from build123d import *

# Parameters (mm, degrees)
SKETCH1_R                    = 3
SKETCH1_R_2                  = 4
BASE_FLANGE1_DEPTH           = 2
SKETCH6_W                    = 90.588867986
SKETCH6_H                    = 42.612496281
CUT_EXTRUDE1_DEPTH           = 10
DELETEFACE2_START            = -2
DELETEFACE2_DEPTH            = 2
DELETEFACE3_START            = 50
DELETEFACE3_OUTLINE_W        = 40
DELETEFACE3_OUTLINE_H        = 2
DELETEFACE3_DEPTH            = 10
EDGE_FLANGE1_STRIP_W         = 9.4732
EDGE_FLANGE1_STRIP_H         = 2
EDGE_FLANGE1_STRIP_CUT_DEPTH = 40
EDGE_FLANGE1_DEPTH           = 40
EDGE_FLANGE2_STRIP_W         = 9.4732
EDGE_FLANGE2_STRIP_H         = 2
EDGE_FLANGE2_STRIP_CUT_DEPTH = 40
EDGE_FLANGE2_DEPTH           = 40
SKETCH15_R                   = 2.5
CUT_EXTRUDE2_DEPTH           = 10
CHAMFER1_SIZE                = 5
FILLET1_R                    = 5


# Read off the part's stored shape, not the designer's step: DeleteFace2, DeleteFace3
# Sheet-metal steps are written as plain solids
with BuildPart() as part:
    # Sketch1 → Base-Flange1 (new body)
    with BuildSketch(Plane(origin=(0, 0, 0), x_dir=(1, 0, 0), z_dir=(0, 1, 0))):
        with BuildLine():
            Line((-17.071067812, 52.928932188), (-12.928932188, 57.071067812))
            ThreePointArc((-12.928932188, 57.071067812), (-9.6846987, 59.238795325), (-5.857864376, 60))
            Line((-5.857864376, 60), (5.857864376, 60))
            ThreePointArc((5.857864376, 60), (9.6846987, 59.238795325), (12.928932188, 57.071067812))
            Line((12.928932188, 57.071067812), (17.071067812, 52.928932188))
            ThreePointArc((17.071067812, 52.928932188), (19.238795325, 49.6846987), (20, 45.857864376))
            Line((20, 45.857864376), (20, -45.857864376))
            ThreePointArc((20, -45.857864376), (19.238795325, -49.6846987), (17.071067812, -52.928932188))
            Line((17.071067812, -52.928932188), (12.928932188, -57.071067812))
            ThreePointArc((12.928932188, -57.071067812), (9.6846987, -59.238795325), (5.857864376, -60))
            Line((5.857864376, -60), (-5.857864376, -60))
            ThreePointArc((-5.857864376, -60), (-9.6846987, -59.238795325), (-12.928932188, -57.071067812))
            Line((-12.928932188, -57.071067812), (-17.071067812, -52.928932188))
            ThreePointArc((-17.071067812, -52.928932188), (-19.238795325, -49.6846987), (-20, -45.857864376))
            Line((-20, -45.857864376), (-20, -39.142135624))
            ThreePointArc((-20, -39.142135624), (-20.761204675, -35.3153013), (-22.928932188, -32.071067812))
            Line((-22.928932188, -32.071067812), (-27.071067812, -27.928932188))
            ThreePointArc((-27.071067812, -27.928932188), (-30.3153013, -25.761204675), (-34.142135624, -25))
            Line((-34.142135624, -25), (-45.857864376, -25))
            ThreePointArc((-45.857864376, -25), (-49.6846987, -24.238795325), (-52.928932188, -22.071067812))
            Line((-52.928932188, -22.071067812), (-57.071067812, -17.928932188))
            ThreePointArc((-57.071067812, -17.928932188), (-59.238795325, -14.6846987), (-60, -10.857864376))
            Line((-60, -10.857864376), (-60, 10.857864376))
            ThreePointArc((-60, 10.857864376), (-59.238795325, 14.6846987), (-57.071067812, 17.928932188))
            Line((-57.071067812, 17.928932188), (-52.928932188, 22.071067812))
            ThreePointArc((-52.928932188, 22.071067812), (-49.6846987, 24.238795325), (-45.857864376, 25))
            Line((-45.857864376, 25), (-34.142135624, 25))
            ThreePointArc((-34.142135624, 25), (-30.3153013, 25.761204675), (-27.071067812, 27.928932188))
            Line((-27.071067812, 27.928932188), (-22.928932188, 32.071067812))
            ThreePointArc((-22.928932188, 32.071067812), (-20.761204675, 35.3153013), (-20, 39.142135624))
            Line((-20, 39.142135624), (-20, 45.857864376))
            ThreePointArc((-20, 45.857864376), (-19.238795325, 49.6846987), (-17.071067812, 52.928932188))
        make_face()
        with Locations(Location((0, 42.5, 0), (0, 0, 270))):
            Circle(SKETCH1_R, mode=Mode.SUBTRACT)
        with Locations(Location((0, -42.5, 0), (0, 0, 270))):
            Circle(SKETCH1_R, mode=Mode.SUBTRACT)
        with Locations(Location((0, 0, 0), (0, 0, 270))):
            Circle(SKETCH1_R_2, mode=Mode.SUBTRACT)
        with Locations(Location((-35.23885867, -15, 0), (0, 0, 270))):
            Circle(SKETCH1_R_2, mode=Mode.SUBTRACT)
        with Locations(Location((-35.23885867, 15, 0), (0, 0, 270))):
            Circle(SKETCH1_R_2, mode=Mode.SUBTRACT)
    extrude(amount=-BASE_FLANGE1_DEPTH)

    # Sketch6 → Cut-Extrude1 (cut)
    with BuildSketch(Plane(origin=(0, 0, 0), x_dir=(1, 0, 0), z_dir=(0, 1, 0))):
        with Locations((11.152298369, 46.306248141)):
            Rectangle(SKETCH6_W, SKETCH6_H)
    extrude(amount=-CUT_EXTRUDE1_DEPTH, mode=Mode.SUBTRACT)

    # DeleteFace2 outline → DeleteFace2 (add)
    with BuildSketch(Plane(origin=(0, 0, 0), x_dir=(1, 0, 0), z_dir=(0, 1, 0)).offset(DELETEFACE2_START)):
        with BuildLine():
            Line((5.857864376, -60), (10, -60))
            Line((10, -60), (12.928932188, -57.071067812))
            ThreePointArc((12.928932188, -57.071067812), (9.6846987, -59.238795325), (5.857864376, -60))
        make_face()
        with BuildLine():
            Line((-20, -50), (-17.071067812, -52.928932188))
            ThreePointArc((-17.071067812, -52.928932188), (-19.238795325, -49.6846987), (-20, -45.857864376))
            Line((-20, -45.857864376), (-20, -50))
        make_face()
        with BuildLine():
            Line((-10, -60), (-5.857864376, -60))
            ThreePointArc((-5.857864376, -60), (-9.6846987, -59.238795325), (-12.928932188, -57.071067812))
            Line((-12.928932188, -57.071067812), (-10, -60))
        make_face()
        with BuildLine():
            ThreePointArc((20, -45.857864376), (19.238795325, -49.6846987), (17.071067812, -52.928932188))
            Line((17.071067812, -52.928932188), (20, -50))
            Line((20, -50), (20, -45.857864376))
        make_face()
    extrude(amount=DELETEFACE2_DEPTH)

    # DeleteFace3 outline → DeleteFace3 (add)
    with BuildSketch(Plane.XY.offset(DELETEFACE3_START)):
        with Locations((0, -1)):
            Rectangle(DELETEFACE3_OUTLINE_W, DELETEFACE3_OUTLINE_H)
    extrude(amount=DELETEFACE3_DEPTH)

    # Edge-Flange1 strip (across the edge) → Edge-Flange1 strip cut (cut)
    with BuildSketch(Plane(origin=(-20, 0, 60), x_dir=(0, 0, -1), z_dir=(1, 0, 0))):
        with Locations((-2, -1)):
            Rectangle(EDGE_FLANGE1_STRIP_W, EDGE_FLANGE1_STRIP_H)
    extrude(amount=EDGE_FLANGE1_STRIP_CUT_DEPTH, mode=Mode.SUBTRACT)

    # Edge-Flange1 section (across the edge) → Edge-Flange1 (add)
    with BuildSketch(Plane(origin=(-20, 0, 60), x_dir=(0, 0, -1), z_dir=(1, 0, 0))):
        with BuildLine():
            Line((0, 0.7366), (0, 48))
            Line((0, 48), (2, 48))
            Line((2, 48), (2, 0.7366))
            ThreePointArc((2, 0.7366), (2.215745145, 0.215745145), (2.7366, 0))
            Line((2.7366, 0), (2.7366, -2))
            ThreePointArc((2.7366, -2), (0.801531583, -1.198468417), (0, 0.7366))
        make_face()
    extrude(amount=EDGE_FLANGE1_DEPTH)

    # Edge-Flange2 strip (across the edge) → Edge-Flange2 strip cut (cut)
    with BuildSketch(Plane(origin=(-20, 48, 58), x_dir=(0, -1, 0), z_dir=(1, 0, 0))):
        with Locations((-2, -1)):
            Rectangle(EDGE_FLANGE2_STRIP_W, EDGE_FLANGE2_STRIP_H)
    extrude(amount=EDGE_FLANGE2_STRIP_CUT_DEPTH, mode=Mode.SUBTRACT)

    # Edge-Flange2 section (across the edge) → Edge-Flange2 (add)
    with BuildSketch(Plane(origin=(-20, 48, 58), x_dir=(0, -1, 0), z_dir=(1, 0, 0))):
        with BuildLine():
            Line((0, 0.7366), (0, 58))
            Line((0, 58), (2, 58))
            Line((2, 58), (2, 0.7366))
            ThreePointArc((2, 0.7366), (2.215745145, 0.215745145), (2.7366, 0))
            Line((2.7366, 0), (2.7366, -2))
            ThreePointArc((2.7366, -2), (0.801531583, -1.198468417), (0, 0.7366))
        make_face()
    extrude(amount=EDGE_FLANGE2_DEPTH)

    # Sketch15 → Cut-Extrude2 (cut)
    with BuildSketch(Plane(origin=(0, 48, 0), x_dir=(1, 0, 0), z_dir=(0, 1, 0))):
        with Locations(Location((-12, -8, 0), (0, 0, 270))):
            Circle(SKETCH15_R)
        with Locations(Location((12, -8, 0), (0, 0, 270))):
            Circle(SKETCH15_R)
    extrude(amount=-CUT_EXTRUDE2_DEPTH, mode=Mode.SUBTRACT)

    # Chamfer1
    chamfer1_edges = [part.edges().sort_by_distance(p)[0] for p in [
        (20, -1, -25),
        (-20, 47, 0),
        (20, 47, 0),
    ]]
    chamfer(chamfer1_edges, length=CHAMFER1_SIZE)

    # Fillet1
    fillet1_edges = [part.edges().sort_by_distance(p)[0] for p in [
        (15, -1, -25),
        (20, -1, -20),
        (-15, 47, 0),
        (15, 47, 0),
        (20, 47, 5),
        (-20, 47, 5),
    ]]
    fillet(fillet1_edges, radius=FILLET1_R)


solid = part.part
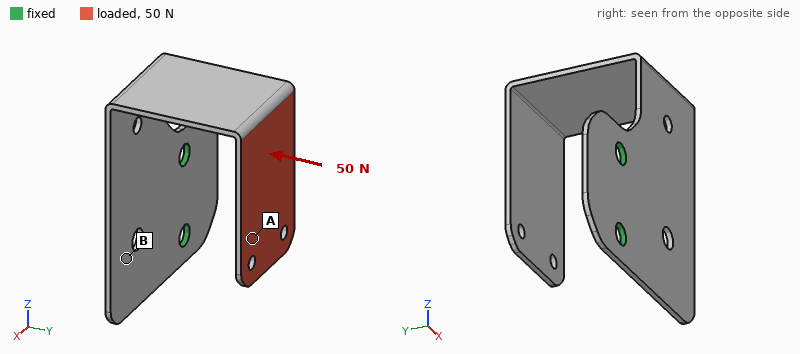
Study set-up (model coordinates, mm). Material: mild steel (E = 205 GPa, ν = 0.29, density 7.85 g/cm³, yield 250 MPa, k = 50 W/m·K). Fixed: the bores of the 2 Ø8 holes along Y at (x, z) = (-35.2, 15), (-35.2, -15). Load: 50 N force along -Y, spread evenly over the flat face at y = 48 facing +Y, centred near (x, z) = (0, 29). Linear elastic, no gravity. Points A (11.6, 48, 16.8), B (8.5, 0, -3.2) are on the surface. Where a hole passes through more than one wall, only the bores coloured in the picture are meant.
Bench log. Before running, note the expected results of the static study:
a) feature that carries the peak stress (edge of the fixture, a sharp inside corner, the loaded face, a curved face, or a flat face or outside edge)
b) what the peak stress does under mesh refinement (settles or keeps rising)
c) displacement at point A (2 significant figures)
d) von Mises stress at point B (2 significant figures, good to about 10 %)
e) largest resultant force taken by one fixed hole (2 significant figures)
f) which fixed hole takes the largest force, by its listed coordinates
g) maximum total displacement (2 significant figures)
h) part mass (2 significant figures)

edge of the fixture
keeps rising
1.0 mm
16 MPa
61 N
(-35.2, 15)
1.3 mm
150 g
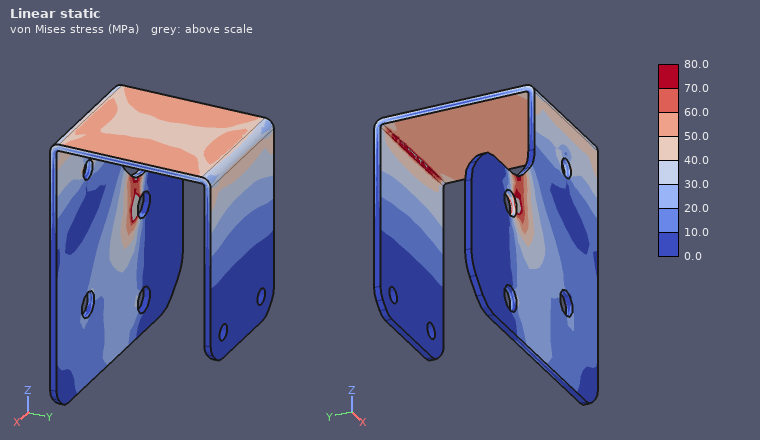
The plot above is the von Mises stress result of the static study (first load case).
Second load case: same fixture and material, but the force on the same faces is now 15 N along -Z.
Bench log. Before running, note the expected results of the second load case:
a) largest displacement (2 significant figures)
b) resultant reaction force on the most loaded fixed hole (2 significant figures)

0.60 mm
22 N
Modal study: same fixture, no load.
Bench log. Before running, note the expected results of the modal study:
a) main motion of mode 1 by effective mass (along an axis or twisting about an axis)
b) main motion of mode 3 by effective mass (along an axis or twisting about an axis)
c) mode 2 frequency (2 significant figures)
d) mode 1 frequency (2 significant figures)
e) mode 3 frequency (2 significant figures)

along Z
along Y
150 Hz
120 Hz
250 Hz
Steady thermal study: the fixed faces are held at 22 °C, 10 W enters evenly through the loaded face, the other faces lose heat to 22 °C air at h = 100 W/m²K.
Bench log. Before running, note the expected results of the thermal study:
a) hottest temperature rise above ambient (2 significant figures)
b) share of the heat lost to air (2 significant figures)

31 K
100 %
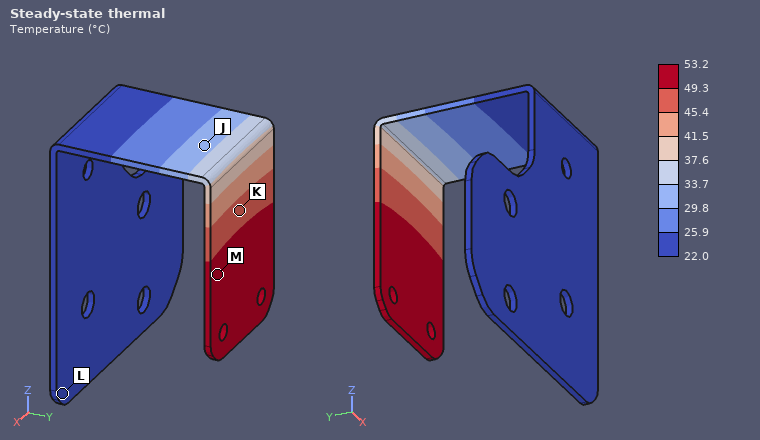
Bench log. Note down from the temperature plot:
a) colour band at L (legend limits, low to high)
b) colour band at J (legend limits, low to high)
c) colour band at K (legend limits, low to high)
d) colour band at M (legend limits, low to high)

22.0 to 25.9 °C
29.8 to 33.7 °C
45.4 to 49.3 °C
49.3 to 53.2 °C
